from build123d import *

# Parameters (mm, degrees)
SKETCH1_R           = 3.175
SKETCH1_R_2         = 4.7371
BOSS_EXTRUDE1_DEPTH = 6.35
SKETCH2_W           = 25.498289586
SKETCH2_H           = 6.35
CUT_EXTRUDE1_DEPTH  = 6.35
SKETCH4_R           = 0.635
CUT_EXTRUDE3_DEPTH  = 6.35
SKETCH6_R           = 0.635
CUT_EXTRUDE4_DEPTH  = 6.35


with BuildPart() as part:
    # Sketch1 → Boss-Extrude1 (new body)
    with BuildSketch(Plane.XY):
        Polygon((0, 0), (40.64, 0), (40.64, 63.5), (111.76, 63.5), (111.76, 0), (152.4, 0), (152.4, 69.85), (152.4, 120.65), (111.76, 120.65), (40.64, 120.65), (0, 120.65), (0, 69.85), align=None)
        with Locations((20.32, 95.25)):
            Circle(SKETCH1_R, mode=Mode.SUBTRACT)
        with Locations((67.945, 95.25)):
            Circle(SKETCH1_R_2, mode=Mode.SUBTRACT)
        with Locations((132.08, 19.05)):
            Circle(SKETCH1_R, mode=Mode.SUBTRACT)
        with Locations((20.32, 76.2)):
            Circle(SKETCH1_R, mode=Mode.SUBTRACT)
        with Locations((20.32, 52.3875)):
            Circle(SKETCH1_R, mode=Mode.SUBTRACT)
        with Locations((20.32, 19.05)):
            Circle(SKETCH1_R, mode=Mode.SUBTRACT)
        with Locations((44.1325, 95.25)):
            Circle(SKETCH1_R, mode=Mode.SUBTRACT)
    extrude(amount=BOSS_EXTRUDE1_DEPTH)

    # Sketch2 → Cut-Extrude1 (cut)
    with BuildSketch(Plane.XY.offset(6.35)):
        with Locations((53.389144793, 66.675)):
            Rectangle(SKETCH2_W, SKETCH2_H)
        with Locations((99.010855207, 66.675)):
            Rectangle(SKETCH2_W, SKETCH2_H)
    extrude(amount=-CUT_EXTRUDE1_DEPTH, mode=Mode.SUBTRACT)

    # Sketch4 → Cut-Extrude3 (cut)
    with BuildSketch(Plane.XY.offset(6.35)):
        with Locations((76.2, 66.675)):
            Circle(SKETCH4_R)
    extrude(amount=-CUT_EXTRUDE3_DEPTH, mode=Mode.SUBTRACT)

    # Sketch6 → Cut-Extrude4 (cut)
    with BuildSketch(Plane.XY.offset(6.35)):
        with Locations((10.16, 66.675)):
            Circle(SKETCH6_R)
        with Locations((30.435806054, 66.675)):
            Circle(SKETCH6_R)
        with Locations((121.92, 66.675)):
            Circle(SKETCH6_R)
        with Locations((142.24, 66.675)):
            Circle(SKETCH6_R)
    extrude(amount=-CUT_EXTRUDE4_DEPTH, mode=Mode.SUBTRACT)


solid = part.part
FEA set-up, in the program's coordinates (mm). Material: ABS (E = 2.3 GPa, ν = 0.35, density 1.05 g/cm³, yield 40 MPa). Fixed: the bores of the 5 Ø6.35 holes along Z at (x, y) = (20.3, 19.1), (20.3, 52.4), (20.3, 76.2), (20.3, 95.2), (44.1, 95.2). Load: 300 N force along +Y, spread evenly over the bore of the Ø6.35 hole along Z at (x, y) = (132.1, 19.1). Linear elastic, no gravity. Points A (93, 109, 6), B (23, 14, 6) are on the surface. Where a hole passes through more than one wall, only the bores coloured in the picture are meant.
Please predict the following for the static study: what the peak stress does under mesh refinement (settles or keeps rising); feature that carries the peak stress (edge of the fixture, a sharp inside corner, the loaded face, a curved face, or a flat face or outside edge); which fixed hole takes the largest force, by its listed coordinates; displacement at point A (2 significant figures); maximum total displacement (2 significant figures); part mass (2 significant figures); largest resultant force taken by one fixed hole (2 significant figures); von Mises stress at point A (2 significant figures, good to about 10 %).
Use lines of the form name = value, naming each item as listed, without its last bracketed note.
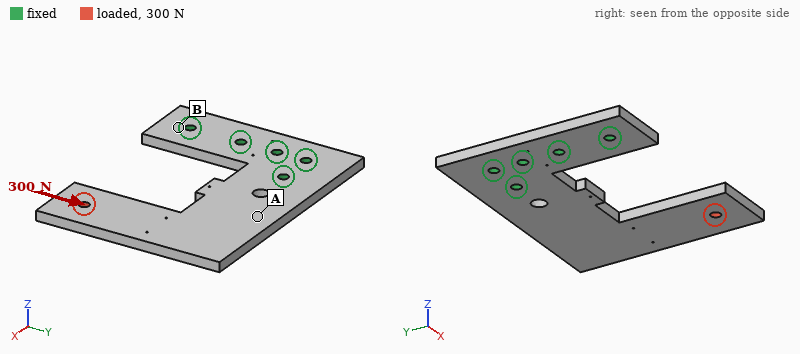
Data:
what the peak stress does under mesh refinement = keeps rising
feature that carries the peak stress = edge of the fixture
which fixed hole takes the largest force, by its listed coordinates = (44.1, 95.2)
displacement at point A = 0.44 mm
maximum total displacement = 1.5 mm
part mass = 89 g
largest resultant force taken by one fixed hole = 700 N
von Mises stress at point A = 2.9 MPa
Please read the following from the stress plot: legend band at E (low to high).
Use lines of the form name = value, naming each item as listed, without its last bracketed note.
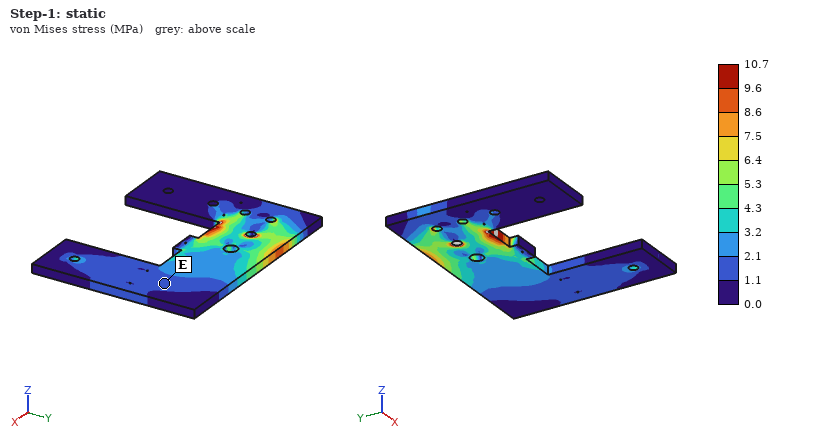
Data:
legend band at E = 1.1 to 2.1 MPa
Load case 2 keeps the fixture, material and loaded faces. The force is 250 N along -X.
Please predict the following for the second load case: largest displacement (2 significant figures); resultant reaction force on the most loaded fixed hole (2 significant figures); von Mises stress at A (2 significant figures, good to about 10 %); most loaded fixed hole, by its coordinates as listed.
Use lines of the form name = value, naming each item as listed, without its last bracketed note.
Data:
largest displacement = 2.0 mm
resultant reaction force on the most loaded fixed hole = 340 N
von Mises stress at A = 2.9 MPa
most loaded fixed hole, by its coordinates as listed = (20.3, 76.2)
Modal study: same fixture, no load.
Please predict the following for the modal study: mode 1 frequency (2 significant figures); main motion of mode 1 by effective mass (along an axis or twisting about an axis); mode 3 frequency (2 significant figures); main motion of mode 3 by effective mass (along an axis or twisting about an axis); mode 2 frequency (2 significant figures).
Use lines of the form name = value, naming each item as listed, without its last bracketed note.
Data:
mode 1 frequency = 73 Hz
main motion of mode 1 by effective mass = along Z
mode 3 frequency = 410 Hz
main motion of mode 3 by effective mass = along Y
mode 2 frequency = 160 Hz
